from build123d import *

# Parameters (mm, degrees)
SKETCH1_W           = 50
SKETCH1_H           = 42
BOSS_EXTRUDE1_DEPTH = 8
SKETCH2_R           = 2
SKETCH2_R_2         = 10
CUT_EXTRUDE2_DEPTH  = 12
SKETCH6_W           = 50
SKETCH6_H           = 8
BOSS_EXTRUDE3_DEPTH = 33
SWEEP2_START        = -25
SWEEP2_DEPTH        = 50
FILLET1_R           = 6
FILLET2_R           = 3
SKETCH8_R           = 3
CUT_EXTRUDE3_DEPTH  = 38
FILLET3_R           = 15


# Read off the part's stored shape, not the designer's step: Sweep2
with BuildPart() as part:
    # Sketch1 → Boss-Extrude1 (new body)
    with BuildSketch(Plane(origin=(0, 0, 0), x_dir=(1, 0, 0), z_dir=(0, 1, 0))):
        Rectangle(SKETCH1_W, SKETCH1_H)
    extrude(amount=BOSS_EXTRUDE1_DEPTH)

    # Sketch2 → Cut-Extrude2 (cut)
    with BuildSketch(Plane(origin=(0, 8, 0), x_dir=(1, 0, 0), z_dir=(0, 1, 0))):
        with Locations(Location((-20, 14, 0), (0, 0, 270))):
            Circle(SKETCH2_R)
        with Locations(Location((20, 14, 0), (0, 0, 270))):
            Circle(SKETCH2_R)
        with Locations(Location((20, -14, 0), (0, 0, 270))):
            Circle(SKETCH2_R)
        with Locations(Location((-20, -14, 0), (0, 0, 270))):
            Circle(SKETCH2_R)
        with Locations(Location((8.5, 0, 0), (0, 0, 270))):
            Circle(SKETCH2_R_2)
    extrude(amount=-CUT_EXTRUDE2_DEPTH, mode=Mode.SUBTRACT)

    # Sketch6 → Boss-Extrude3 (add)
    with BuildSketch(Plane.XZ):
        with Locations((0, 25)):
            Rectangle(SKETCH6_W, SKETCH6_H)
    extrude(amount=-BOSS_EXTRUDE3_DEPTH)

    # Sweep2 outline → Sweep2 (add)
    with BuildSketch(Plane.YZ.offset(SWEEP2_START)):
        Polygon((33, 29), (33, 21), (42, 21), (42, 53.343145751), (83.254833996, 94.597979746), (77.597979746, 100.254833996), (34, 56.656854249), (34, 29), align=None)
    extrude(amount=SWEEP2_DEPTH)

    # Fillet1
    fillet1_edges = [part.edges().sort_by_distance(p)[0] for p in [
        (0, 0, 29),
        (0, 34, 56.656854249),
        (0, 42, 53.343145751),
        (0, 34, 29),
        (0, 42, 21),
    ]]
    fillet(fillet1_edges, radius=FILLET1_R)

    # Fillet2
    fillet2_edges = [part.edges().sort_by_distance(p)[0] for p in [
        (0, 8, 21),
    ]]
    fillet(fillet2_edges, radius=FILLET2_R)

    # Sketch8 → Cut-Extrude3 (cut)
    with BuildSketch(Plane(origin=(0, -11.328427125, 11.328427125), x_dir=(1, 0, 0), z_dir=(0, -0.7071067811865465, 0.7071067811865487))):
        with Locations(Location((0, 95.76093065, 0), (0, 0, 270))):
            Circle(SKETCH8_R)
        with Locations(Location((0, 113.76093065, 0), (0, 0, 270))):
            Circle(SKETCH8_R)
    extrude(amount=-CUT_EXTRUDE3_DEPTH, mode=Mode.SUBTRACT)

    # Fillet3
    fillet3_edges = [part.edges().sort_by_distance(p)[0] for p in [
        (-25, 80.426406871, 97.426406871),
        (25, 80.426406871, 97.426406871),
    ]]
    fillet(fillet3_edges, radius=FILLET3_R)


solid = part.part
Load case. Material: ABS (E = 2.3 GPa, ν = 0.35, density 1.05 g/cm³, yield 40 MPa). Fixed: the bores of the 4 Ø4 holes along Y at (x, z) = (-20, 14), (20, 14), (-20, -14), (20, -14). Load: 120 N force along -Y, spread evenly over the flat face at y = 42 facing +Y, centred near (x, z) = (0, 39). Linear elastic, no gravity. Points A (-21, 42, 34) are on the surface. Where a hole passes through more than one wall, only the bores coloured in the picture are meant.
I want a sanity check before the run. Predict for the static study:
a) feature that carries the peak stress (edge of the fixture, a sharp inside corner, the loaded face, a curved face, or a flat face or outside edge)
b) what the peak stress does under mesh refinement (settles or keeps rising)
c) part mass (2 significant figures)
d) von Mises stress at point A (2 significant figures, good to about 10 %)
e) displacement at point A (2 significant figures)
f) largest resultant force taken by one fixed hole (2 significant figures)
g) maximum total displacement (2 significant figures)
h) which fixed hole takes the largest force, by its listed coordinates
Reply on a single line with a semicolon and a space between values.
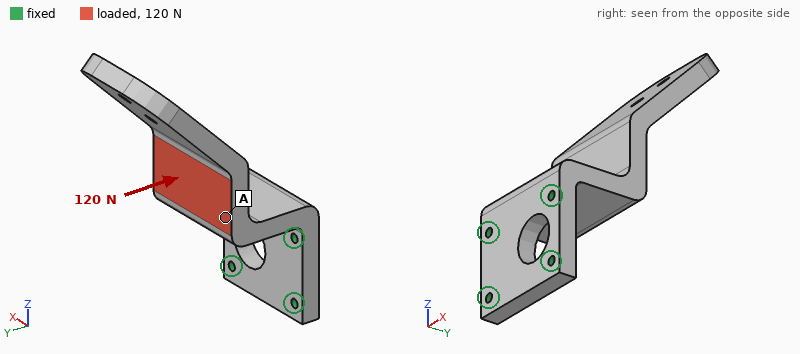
edge of the fixture; keeps rising; 67 g; 1.3 MPa; 0.46 mm; 80 N; 1.6 mm; (-20, 14)
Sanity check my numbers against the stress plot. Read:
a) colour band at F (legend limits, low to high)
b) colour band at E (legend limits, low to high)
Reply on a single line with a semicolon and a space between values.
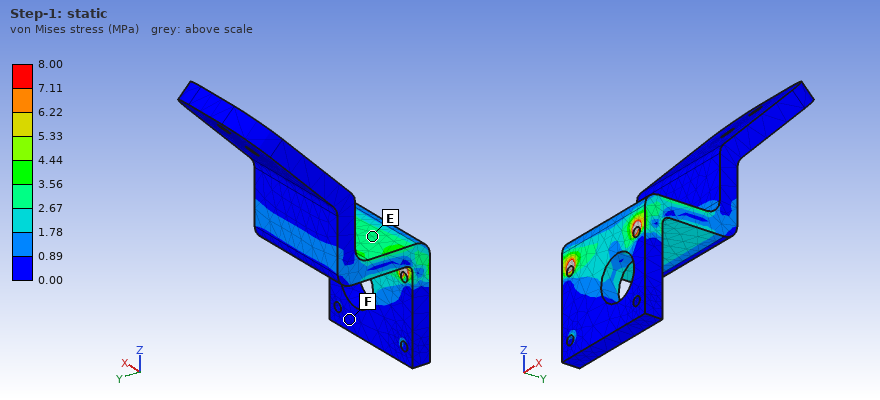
0.00 to 0.89 MPa; 2.67 to 3.56 MPa
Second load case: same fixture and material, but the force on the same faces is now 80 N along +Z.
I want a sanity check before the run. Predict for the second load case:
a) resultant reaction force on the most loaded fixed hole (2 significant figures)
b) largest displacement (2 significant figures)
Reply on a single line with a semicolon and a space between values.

39 N; 1.7 mm
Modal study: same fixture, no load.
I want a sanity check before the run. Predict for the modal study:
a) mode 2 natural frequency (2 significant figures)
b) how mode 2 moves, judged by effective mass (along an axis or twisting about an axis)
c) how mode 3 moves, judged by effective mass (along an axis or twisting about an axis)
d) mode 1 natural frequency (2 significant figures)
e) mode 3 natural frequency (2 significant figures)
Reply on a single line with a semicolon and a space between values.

390 Hz; along X; along Z; 140 Hz; 750 Hz
